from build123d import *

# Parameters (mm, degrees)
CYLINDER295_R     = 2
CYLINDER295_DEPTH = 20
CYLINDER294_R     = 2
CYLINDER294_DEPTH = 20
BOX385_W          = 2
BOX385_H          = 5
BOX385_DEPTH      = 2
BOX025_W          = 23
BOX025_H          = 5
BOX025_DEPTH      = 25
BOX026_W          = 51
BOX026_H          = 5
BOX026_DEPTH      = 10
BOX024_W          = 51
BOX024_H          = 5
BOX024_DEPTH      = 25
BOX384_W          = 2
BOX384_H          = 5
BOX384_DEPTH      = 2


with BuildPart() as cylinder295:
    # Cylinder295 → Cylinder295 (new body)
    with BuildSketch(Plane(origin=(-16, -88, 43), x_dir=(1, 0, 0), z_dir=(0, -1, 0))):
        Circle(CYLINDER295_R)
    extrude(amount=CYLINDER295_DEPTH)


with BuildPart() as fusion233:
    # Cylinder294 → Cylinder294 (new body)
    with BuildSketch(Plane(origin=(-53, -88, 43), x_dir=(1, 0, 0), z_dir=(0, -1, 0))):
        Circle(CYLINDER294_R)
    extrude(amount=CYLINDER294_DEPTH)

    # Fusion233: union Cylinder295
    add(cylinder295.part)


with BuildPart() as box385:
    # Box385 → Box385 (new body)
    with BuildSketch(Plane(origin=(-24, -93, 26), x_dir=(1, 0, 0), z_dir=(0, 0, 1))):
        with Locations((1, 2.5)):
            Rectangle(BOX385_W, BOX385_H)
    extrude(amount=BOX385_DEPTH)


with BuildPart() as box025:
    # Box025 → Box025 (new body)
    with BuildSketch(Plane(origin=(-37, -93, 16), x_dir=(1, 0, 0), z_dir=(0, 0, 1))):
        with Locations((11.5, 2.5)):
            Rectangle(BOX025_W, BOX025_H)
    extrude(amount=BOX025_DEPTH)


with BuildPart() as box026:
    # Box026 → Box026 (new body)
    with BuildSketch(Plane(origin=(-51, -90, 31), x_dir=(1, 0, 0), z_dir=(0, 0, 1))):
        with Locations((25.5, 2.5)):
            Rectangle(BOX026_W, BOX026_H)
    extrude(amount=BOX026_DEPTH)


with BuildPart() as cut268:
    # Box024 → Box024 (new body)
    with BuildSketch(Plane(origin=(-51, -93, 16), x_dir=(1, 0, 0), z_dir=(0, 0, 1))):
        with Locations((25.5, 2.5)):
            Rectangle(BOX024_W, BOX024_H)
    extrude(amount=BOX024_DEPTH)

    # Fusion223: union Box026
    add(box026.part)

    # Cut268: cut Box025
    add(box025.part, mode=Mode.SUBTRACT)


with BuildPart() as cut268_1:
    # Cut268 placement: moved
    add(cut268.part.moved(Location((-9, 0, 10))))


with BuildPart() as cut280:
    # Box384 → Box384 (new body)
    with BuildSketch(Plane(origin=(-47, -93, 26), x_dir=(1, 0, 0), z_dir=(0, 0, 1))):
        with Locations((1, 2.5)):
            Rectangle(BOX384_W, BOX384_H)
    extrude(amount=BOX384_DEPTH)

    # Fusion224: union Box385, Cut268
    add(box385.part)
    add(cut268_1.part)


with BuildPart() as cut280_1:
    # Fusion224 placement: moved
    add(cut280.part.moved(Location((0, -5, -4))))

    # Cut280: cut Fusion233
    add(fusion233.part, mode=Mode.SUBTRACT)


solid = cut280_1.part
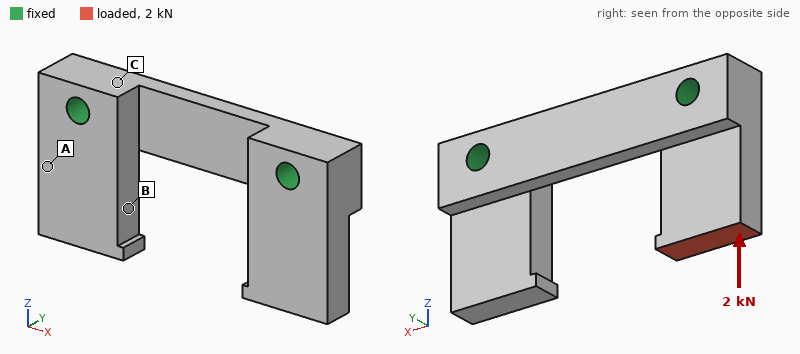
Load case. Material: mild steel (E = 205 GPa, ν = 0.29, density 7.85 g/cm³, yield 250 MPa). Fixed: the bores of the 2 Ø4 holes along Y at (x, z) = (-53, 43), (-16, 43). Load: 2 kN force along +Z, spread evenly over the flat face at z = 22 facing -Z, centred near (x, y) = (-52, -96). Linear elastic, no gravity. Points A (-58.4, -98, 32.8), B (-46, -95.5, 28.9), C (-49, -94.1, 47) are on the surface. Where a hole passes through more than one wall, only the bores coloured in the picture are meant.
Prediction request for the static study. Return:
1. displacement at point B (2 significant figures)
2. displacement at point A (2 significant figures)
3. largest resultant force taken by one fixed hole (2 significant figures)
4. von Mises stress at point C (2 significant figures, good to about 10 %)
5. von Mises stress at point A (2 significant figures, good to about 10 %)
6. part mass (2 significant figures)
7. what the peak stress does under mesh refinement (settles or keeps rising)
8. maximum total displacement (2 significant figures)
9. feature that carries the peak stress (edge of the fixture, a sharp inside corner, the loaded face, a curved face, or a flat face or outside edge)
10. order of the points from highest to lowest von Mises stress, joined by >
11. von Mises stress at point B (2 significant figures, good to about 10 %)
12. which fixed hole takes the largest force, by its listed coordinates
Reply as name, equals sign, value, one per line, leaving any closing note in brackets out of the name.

displacement at point B = 3.1 µm
displacement at point A = 1.9 µm
largest resultant force taken by one fixed hole = 2.0 kN
von Mises stress at point C = 9.7 MPa
von Mises stress at point A = 23 MPa
part mass = 38 g
what the peak stress does under mesh refinement = keeps rising
maximum total displacement = 5.6 µm
feature that carries the peak stress = edge of the fixture
order of the points from highest to lowest von Mises stress, joined by > = B > A > C
von Mises stress at point B = 37 MPa
which fixed hole takes the largest force, by its listed coordinates = (-53, 43)
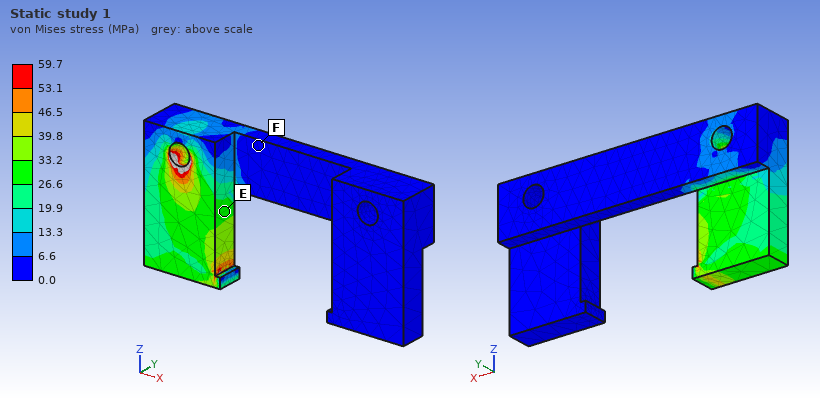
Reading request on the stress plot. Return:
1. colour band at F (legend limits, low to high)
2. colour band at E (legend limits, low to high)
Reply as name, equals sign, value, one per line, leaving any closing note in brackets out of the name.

colour band at F = 0.0 to 6.6 MPa
colour band at E = 26.6 to 33.2 MPa
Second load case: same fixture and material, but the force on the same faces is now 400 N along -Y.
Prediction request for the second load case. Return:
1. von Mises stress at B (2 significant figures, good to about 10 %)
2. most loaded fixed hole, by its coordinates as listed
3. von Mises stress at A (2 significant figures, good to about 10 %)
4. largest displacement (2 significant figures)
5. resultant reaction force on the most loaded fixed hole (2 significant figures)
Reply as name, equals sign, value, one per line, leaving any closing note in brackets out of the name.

von Mises stress at B = 24 MPa
most loaded fixed hole, by its coordinates as listed = (-53, 43)
von Mises stress at A = 73 MPa
largest displacement = 28 µm
resultant reaction force on the most loaded fixed hole = 400 N
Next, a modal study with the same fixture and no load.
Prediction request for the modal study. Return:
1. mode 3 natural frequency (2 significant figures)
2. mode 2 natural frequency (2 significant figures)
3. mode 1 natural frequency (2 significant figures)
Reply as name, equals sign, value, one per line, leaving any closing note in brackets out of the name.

mode 3 natural frequency = 16 kHz
mode 2 natural frequency = 12 kHz
mode 1 natural frequency = 12 kHz
